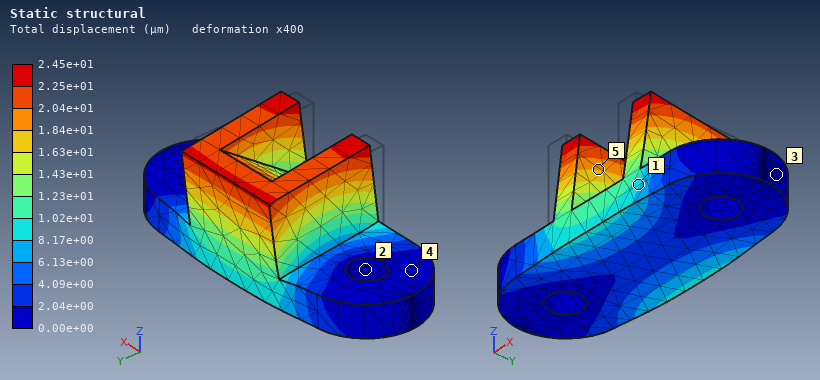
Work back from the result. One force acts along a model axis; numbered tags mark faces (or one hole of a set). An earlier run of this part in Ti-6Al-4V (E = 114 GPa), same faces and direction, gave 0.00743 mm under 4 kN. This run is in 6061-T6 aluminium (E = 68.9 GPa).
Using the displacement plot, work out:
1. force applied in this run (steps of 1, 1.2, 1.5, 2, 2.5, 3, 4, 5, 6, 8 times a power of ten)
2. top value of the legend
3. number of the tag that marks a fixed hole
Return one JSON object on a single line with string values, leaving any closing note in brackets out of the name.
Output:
{"force applied in this run": "8 kN", "top value of the legend": "2.45e+01 µm", "number of the tag that marks a fixed hole": "2"}
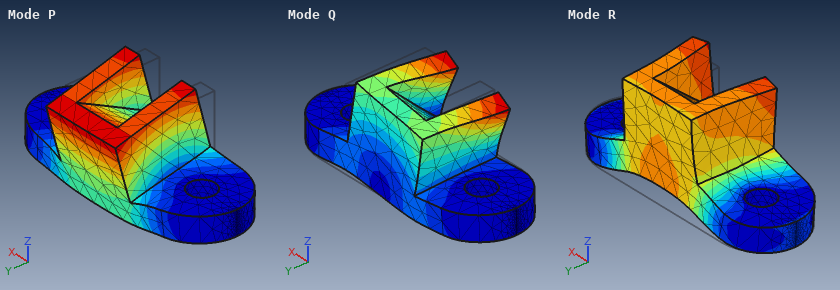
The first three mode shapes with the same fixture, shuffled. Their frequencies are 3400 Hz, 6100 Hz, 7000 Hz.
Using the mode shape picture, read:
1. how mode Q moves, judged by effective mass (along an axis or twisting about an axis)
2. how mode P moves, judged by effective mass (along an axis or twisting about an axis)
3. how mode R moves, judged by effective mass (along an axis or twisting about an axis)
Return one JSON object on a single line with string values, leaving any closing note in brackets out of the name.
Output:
{"how mode Q moves, judged by effective mass": "along X", "how mode P moves, judged by effective mass": "along Y", "how mode R moves, judged by effective mass": "along Z"}
